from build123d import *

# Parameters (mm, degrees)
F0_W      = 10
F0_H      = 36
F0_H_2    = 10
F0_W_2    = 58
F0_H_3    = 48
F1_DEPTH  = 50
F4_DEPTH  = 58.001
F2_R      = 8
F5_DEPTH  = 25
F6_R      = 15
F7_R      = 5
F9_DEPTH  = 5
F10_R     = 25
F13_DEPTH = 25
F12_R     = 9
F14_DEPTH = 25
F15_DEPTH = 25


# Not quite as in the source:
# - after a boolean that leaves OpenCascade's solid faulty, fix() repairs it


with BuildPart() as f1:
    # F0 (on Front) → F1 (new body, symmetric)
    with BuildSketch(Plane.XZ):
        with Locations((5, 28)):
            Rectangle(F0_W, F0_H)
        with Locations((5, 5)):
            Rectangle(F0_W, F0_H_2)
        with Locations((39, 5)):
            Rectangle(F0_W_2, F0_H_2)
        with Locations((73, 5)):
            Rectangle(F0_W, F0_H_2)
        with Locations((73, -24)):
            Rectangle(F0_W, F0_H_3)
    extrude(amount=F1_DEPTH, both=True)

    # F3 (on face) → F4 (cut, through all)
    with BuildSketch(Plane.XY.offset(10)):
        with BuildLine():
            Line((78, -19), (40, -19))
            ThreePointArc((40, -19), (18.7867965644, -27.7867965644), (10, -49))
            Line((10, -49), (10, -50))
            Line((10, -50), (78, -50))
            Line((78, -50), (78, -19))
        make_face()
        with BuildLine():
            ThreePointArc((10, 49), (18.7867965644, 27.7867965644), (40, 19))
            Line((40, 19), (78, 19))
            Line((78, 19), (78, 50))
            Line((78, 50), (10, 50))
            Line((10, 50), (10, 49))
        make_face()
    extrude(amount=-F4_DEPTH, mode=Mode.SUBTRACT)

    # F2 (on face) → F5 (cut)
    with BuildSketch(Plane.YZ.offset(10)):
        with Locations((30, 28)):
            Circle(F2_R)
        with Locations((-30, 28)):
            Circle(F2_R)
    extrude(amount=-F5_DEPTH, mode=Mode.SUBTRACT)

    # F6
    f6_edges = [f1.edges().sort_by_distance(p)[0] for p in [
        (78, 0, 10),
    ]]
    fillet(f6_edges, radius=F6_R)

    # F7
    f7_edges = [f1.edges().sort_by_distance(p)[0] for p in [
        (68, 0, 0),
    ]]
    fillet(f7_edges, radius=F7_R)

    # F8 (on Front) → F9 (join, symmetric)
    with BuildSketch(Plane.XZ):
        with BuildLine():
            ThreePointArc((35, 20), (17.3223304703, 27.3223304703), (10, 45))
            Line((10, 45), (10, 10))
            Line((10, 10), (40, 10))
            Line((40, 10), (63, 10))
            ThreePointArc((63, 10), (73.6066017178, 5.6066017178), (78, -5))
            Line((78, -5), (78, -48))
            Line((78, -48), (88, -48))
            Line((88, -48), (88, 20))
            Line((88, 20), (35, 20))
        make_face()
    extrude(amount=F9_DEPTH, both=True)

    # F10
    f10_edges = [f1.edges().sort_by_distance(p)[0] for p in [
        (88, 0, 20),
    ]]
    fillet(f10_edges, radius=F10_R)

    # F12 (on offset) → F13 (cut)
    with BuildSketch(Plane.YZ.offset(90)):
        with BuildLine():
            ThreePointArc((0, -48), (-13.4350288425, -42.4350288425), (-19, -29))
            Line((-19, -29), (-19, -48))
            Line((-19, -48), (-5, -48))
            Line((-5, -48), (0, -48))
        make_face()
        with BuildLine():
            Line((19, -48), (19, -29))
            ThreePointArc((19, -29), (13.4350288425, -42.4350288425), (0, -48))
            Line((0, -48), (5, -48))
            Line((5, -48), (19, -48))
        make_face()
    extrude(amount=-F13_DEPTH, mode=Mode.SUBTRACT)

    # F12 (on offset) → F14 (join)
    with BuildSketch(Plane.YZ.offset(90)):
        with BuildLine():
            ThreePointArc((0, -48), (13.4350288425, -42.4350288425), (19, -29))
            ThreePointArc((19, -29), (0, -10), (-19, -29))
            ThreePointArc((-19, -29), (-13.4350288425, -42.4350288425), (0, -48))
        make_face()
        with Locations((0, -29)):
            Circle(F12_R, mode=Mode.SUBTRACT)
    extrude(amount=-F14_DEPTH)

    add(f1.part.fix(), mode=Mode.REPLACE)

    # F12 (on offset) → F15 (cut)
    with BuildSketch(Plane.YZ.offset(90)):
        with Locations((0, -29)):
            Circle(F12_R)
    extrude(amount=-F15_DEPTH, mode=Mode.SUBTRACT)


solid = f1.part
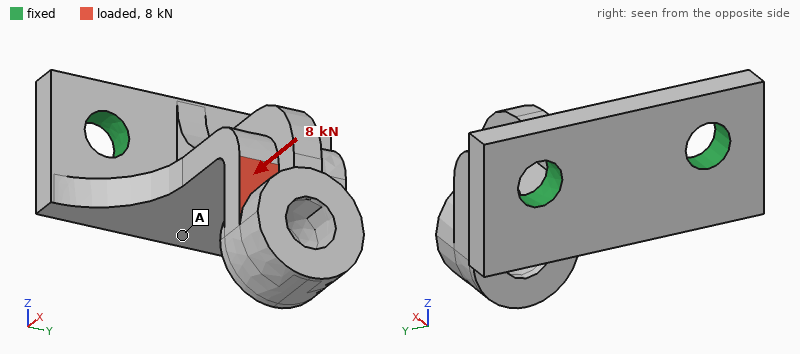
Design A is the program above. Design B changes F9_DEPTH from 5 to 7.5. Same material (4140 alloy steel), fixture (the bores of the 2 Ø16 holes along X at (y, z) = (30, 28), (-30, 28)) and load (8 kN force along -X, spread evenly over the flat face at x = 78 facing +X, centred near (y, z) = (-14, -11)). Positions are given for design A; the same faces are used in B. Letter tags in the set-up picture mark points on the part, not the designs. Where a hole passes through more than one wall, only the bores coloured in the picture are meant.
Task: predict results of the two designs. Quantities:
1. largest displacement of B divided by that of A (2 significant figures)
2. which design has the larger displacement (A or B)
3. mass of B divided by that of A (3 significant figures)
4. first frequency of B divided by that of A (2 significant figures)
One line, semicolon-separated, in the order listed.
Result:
0.88; A; 1.05; 1.1
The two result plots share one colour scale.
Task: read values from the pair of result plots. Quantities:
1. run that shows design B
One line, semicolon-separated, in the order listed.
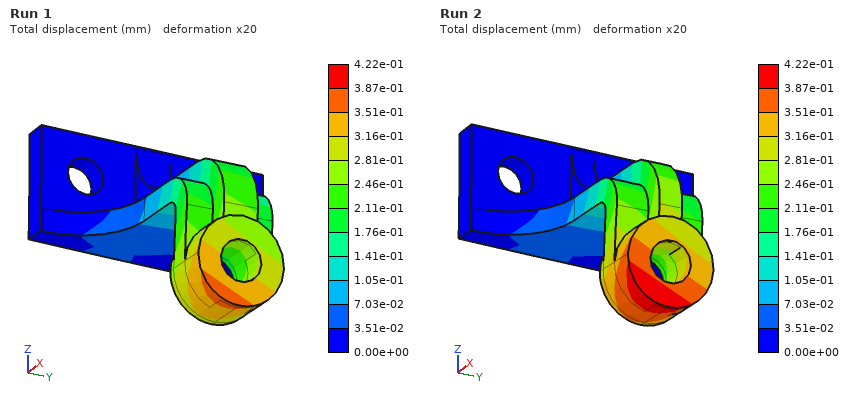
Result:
Run 1
